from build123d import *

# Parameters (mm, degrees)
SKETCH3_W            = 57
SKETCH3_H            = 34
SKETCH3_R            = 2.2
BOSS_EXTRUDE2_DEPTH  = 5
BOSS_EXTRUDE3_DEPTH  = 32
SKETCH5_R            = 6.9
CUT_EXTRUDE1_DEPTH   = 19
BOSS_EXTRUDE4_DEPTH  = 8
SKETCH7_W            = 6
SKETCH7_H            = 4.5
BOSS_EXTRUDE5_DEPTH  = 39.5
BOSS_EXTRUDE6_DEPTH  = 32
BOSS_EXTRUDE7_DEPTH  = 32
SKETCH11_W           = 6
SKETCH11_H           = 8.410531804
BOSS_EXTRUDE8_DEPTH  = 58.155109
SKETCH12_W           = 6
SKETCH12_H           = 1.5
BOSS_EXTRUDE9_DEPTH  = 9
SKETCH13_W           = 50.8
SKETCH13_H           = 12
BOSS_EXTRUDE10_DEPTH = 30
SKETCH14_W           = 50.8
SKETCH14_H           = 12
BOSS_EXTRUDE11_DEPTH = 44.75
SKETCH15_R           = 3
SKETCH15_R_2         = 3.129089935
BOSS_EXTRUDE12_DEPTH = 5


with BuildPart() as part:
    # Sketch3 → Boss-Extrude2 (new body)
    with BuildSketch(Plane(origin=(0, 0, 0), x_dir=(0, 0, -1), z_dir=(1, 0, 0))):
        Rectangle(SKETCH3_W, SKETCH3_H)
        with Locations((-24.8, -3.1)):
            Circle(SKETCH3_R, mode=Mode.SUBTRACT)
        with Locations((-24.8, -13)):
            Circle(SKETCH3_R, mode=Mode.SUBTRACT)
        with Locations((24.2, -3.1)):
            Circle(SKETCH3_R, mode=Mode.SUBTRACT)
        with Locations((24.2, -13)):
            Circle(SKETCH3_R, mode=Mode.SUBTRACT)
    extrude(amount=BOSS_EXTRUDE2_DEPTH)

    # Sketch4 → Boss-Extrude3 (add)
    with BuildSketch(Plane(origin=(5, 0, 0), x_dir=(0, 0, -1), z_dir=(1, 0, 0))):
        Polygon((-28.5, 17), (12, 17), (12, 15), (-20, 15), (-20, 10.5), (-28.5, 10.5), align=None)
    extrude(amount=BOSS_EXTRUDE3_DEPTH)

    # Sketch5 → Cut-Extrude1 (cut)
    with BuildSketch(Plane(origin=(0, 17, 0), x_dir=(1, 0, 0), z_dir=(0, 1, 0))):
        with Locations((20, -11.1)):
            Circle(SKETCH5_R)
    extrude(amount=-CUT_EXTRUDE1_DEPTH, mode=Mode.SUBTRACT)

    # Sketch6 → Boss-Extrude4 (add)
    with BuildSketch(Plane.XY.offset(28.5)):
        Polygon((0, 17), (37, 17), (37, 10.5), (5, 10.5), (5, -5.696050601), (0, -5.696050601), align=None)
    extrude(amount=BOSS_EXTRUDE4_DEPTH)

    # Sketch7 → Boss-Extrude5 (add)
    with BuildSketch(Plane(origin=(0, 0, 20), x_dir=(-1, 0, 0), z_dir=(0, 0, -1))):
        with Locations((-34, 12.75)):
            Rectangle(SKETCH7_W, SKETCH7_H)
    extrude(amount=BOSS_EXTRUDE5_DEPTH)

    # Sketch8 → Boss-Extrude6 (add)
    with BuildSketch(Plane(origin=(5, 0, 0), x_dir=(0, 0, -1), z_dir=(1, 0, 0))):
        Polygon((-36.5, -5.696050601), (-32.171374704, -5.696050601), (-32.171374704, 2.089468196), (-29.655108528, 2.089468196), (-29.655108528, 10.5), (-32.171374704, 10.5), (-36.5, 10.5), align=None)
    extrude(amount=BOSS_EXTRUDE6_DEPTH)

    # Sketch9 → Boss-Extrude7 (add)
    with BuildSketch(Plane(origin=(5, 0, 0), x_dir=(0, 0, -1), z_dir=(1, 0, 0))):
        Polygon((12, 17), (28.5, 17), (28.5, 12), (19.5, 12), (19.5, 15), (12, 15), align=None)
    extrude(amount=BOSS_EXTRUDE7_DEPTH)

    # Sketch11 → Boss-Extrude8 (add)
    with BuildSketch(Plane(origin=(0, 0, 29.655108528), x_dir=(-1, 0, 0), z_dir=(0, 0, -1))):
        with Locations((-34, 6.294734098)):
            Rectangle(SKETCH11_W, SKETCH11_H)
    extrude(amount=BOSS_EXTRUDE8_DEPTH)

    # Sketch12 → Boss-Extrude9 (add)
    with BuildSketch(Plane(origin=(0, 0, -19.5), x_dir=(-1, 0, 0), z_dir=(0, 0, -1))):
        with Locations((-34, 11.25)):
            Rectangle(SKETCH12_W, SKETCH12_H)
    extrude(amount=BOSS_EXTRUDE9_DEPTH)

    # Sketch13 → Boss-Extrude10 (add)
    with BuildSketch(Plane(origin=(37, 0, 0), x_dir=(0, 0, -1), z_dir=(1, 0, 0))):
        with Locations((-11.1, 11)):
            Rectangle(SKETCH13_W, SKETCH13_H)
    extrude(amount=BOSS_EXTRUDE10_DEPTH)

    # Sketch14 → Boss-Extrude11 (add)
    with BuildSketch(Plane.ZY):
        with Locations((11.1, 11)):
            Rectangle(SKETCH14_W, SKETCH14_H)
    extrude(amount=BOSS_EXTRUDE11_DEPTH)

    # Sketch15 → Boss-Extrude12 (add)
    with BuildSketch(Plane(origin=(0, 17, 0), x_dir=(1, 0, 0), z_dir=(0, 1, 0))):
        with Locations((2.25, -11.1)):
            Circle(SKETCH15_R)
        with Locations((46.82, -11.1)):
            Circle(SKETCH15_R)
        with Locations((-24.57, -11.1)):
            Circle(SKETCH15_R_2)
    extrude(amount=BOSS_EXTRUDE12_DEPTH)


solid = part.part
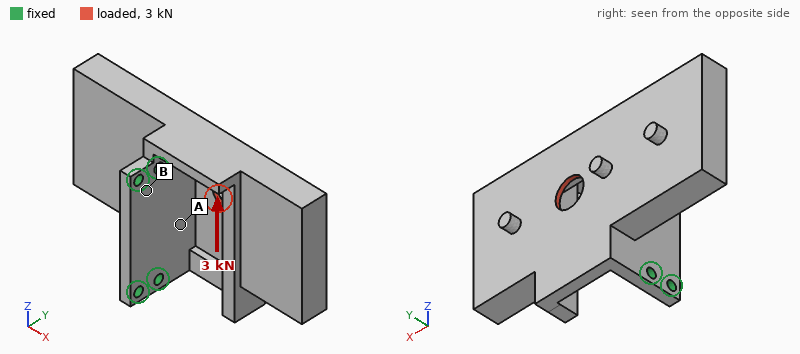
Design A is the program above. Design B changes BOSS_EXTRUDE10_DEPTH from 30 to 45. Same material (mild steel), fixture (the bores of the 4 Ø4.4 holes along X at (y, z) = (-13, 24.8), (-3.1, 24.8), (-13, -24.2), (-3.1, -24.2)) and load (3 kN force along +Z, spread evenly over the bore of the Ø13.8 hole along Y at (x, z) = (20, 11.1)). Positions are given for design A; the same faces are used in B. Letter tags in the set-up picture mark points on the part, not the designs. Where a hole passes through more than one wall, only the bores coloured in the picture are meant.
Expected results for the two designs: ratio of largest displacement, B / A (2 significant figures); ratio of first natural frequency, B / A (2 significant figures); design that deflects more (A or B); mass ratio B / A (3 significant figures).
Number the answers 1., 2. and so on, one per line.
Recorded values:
1. 1.2
2. 0.77
3. B
4. 1.13
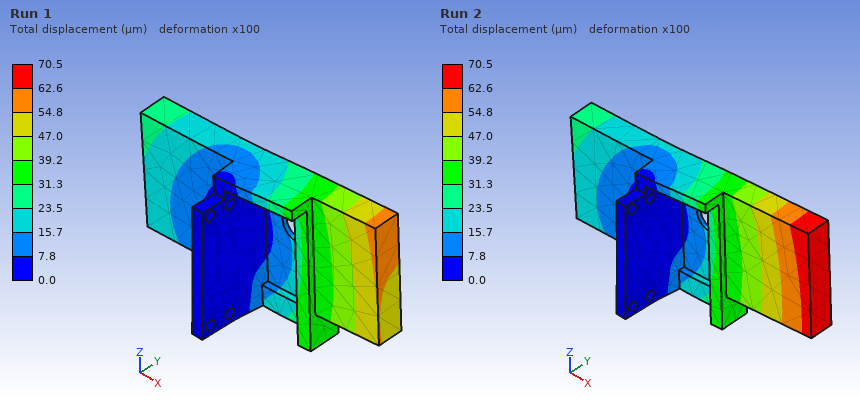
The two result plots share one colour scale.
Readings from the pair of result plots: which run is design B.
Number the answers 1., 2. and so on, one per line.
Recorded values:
1. Run 2
